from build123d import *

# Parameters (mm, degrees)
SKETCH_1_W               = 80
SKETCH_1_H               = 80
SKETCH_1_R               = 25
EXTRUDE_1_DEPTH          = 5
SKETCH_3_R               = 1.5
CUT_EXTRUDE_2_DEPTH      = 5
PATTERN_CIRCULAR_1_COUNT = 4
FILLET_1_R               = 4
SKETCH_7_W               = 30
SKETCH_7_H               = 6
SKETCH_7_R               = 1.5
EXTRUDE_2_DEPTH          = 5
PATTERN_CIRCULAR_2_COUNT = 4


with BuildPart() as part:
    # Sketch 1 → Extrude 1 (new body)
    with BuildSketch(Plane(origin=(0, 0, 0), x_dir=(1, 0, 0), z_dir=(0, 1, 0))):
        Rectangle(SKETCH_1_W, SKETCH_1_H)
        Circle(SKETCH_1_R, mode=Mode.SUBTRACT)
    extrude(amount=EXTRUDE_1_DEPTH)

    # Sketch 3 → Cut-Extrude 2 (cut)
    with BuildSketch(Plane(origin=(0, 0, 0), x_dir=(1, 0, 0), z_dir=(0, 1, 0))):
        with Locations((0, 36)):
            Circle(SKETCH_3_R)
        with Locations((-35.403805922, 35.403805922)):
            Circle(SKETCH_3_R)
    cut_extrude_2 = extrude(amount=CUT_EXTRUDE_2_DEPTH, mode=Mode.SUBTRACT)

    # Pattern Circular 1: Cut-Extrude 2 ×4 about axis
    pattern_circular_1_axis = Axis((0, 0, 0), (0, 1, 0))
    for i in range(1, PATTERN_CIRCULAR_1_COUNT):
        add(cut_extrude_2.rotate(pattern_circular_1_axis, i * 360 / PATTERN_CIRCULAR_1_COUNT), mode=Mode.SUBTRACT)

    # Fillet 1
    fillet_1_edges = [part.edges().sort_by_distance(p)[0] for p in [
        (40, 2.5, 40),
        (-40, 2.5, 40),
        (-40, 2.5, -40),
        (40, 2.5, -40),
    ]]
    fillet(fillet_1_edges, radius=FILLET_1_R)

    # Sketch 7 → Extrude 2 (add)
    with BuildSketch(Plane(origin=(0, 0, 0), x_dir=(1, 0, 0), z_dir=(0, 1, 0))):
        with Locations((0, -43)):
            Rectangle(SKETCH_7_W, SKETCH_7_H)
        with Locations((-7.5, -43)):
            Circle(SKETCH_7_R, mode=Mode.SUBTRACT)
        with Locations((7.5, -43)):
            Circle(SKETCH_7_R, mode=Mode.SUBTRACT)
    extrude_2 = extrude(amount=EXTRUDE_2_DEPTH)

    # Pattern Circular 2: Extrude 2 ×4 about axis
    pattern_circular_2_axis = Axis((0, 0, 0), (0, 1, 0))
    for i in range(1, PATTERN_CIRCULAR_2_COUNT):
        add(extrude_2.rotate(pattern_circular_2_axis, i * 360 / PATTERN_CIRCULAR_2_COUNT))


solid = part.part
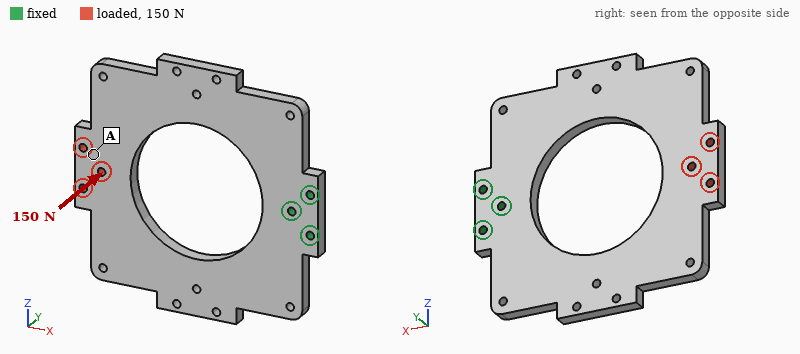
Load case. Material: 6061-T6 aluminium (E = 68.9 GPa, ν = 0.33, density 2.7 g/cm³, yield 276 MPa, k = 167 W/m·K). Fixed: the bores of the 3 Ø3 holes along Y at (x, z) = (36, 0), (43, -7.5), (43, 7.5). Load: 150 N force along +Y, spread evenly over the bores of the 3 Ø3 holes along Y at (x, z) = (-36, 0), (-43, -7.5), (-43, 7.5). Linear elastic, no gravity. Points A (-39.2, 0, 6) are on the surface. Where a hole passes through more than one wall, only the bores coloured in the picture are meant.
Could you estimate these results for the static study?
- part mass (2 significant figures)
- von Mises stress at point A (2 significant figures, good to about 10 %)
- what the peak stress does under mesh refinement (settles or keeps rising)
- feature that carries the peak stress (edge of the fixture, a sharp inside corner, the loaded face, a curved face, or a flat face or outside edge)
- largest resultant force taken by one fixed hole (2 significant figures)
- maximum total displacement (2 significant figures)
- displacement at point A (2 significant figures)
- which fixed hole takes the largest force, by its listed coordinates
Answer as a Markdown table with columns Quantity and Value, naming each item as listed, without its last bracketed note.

| Quantity | Value |
|---|---|
| part mass | 68 g |
| von Mises stress at point A | 13 MPa |
| what the peak stress does under mesh refinement | keeps rising |
| feature that carries the peak stress | edge of the fixture |
| largest resultant force taken by one fixed hole | 760 N |
| maximum total displacement | 1.2 mm |
| displacement at point A | 1.0 mm |
| which fixed hole takes the largest force, by its listed coordinates | (36, 0) |
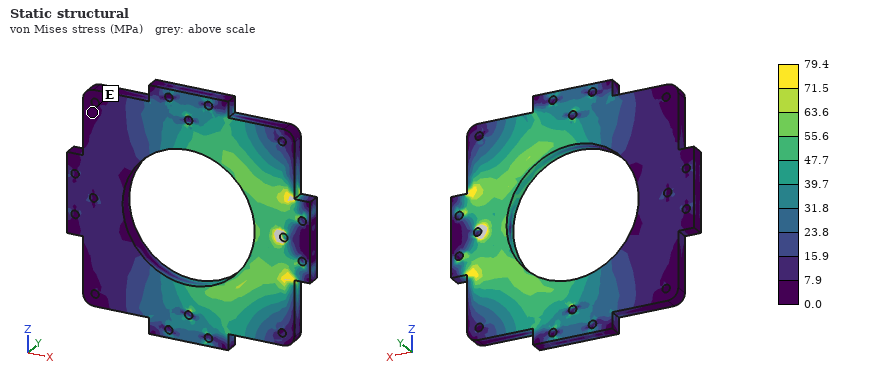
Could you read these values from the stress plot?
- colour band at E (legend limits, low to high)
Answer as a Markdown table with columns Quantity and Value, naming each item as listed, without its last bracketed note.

| Quantity | Value |
|---|---|
| colour band at E | 0.0 to 7.9 MPa |
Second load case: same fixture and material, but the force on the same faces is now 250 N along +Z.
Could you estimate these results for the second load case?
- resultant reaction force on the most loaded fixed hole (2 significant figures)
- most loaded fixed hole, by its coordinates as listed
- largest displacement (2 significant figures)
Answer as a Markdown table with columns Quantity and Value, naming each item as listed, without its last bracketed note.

| Quantity | Value |
|---|---|
| resultant reaction force on the most loaded fixed hole | 1.1 kN |
| most loaded fixed hole, by its coordinates as listed | (36, 0) |
| largest displacement | 77 µm |
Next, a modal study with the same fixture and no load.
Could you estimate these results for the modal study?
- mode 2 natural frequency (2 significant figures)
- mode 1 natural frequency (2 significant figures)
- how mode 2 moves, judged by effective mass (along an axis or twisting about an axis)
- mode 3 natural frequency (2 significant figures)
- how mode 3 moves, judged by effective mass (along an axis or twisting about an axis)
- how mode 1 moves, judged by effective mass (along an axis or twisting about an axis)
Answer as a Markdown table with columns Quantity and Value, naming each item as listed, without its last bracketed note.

| Quantity | Value |
|---|---|
| mode 2 natural frequency | 810 Hz |
| mode 1 natural frequency | 420 Hz |
| how mode 2 moves, judged by effective mass | twisting about X |
| mode 3 natural frequency | 1700 Hz |
| how mode 3 moves, judged by effective mass | along Z |
| how mode 1 moves, judged by effective mass | along Y |
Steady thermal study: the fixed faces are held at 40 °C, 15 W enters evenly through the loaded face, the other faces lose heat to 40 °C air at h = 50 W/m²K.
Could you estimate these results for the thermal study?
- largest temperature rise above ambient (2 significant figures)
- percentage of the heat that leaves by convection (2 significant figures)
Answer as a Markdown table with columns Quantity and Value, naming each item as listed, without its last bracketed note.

| Quantity | Value |
|---|---|
| largest temperature rise above ambient | 31 K |
| percentage of the heat that leaves by convection | 55 % |
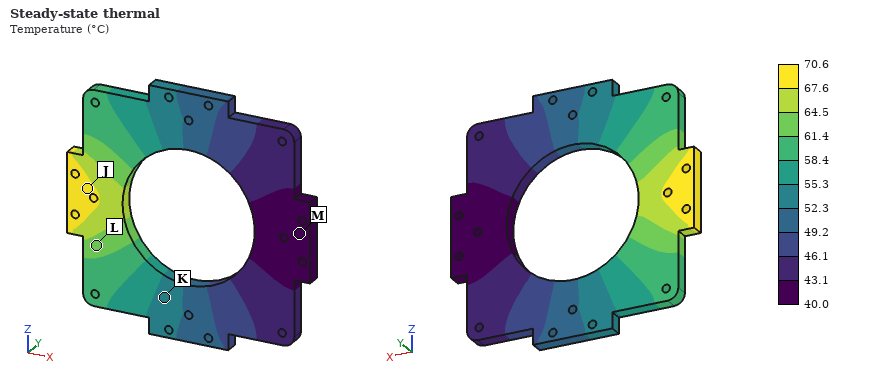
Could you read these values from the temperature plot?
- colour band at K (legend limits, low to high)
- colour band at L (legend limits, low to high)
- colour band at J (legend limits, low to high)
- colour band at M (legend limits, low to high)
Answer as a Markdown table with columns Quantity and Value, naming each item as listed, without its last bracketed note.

| Quantity | Value |
|---|---|
| colour band at K | 52.3 to 55.3 °C |
| colour band at L | 61.4 to 64.5 °C |
| colour band at J | 67.6 to 70.6 °C |
| colour band at M | 40.0 to 43.1 °C |
